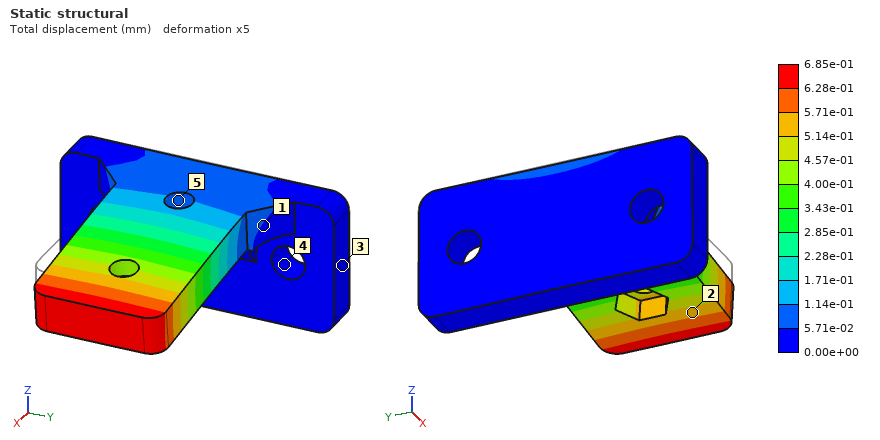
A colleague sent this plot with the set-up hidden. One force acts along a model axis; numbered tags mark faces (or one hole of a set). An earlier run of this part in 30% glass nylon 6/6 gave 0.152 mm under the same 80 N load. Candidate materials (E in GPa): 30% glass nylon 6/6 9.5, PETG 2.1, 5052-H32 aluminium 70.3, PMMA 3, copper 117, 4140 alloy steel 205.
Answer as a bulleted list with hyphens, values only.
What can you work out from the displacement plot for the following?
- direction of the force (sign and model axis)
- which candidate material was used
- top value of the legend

- -Z
- PETG
- 6.85e-01 mm
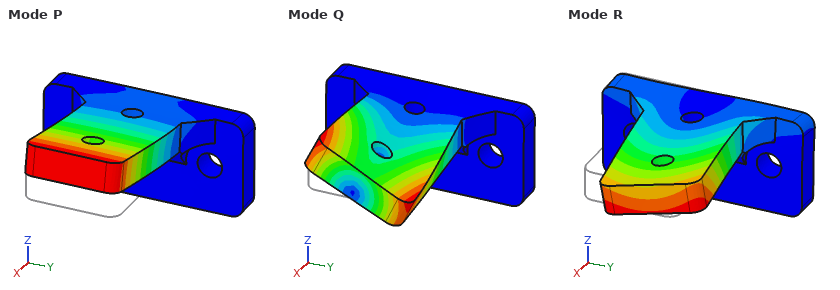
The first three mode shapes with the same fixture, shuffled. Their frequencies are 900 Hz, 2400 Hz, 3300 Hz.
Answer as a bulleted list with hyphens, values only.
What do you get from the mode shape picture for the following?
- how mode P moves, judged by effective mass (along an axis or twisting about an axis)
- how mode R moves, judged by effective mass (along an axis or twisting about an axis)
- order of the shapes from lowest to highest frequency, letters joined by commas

- along Z
- along Y
- P, R, Q
